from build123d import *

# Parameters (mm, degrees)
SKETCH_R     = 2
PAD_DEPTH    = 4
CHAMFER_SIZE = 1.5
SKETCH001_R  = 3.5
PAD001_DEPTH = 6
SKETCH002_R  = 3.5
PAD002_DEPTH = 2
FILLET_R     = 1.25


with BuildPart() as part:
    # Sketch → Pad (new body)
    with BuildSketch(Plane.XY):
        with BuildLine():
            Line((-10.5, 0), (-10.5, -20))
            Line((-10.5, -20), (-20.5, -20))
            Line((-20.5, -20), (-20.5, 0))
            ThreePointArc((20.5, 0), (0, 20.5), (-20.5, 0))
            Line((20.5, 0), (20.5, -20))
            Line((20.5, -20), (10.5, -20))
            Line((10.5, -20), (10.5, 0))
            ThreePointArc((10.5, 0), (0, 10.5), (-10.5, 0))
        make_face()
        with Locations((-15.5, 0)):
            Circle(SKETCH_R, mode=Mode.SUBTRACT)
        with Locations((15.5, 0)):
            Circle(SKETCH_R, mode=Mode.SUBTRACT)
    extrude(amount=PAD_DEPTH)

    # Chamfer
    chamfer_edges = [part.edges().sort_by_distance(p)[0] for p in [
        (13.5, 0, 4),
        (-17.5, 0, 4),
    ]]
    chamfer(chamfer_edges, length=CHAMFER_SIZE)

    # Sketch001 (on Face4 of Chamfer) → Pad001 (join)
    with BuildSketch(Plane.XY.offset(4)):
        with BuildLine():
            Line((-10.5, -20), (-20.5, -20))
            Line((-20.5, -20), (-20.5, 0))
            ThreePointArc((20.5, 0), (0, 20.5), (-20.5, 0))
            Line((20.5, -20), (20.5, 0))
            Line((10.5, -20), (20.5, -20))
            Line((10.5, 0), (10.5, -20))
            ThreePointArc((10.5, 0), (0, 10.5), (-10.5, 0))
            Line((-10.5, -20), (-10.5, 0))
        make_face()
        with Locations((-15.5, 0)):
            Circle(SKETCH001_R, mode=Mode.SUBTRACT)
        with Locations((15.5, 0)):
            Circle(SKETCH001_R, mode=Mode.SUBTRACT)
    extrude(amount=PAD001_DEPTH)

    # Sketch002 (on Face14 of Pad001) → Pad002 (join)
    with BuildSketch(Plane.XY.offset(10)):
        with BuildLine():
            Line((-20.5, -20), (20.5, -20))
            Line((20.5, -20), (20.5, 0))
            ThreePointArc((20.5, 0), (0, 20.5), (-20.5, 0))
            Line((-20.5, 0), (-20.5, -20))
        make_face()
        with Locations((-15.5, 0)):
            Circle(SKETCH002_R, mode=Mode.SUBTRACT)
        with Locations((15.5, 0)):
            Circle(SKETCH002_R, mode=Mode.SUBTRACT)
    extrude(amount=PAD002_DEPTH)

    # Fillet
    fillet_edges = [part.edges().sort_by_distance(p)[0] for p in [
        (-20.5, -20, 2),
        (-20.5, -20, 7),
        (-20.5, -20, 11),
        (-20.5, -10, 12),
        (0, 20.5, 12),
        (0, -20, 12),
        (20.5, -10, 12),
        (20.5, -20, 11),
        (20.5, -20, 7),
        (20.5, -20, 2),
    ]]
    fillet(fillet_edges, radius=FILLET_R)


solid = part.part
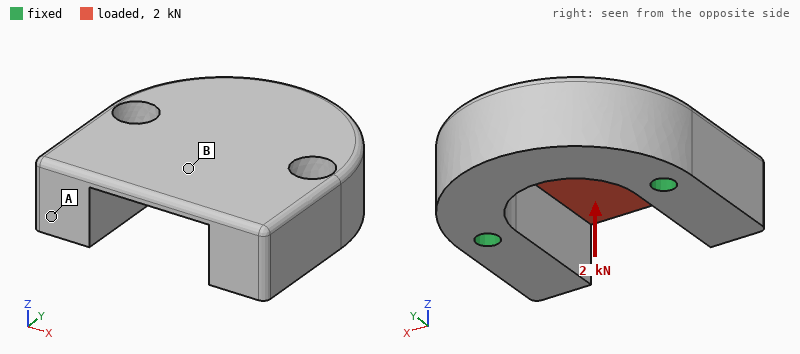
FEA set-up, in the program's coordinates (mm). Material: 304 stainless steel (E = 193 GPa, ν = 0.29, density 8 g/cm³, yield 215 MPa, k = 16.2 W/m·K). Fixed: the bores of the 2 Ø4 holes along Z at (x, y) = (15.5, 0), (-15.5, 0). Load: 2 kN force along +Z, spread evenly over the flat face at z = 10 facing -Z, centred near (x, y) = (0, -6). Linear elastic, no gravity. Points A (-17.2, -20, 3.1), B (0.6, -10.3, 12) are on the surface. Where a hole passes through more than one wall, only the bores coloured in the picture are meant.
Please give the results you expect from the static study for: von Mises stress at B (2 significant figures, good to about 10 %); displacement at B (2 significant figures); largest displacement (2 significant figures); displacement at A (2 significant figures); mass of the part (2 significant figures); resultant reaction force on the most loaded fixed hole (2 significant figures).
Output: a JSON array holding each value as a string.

["110 MPa", "35 µm", "50 µm", "21 µm", "88 g", "1.2 kN"]
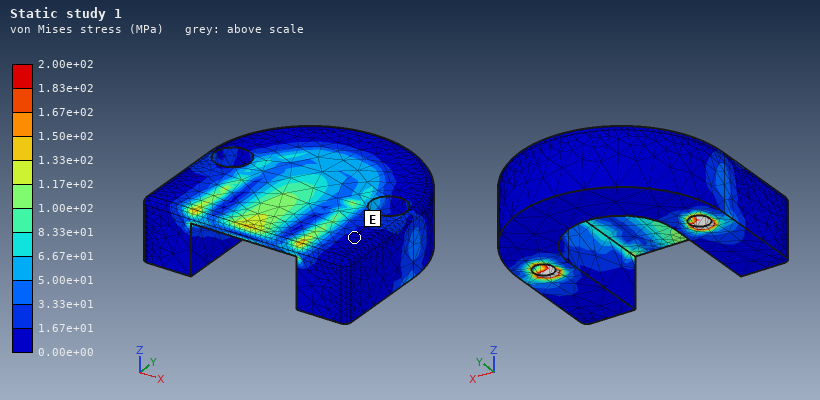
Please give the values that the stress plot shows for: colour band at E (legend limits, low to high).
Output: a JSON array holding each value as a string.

["0.00e+00 to 1.67e+01 MPa"]
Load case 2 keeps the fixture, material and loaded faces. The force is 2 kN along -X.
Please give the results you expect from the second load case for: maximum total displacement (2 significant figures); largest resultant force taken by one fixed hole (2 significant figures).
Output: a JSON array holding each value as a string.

["18 µm", "1.1 kN"]
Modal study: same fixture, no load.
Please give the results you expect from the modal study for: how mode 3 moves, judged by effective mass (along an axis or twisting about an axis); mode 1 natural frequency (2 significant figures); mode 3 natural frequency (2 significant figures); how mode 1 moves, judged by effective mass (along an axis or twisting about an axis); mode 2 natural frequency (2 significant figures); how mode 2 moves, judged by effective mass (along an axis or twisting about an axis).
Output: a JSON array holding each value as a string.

["along Z", "4400 Hz", "14 kHz", "along Y", "8600 Hz", "along X"]
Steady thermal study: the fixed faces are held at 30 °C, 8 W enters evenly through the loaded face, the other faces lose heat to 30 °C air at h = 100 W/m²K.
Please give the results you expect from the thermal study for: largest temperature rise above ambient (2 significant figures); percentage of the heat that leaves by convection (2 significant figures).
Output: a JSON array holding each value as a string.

["34 K", "61 %"]
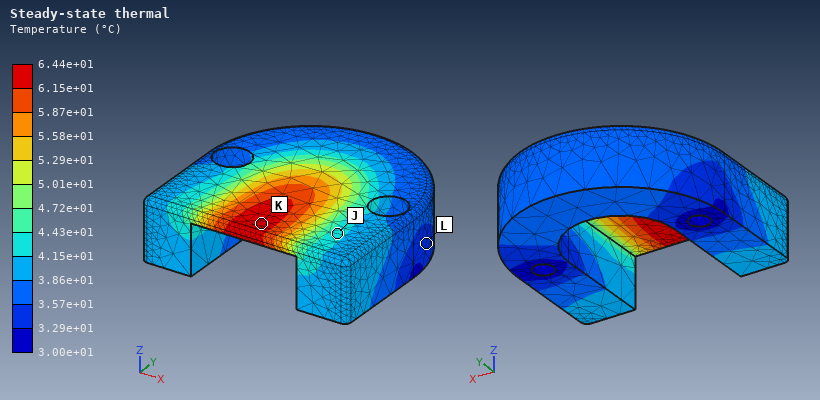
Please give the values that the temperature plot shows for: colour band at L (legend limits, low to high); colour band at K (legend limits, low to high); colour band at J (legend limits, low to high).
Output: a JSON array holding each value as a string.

["3.29e+01 to 3.57e+01 °C", "6.15e+01 to 6.44e+01 °C", "4.15e+01 to 4.43e+01 °C"]
